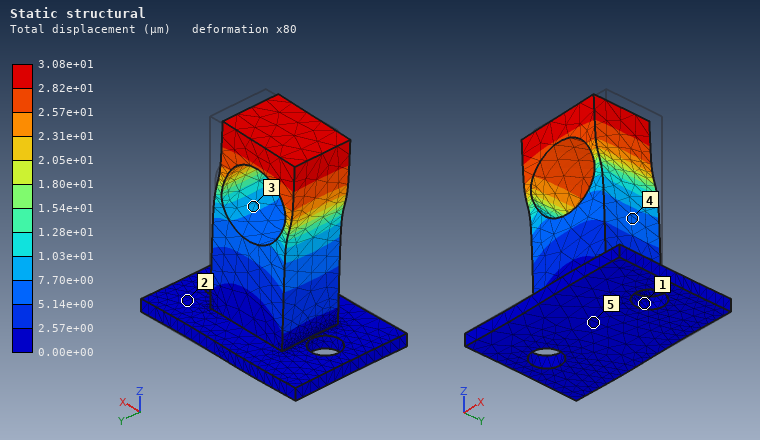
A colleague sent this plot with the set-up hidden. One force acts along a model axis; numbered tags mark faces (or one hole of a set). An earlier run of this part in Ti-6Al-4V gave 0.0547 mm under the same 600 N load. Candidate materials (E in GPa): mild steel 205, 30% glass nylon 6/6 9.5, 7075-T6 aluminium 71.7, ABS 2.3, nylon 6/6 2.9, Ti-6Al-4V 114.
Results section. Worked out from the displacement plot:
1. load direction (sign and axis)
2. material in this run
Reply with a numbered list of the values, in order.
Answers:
1. -X
2. mild steel
